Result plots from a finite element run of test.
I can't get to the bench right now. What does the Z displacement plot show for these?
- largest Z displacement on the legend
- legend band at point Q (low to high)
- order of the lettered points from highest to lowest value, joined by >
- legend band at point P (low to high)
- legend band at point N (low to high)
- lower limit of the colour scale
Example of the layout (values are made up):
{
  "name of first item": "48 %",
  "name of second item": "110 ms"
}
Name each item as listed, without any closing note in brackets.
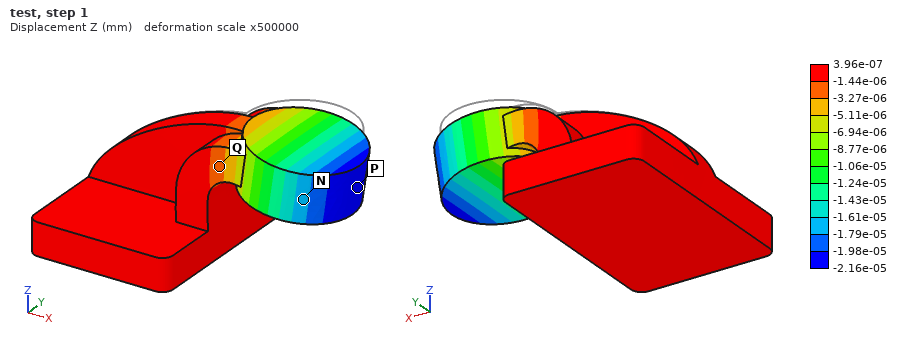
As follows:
{
  "largest Z displacement on the legend": "3.96e-07 mm",
  "legend band at point Q": "-3.27e-06 to -1.44e-06 mm",
  "order of the lettered points from highest to lowest value, joined by >": "Q > N > P",
  "legend band at point P": "-2.16e-05 to -1.98e-05 mm",
  "legend band at point N": "-1.79e-05 to -1.61e-05 mm",
  "lower limit of the colour scale": "-2.16e-05 mm"
}
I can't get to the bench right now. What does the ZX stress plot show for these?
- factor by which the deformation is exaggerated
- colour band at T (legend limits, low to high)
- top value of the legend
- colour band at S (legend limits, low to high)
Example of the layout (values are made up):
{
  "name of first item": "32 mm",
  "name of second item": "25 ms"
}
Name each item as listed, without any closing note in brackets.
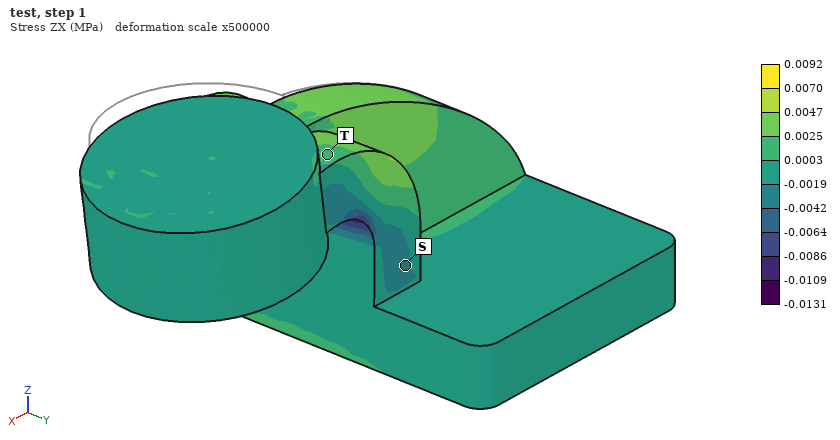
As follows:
{
  "factor by which the deformation is exaggerated": "500000",
  "colour band at T": "0.0003 to 0.0025 MPa",
  "top value of the legend": "0.0092 MPa",
  "colour band at S": "-0.0042 to -0.0019 MPa"
}
